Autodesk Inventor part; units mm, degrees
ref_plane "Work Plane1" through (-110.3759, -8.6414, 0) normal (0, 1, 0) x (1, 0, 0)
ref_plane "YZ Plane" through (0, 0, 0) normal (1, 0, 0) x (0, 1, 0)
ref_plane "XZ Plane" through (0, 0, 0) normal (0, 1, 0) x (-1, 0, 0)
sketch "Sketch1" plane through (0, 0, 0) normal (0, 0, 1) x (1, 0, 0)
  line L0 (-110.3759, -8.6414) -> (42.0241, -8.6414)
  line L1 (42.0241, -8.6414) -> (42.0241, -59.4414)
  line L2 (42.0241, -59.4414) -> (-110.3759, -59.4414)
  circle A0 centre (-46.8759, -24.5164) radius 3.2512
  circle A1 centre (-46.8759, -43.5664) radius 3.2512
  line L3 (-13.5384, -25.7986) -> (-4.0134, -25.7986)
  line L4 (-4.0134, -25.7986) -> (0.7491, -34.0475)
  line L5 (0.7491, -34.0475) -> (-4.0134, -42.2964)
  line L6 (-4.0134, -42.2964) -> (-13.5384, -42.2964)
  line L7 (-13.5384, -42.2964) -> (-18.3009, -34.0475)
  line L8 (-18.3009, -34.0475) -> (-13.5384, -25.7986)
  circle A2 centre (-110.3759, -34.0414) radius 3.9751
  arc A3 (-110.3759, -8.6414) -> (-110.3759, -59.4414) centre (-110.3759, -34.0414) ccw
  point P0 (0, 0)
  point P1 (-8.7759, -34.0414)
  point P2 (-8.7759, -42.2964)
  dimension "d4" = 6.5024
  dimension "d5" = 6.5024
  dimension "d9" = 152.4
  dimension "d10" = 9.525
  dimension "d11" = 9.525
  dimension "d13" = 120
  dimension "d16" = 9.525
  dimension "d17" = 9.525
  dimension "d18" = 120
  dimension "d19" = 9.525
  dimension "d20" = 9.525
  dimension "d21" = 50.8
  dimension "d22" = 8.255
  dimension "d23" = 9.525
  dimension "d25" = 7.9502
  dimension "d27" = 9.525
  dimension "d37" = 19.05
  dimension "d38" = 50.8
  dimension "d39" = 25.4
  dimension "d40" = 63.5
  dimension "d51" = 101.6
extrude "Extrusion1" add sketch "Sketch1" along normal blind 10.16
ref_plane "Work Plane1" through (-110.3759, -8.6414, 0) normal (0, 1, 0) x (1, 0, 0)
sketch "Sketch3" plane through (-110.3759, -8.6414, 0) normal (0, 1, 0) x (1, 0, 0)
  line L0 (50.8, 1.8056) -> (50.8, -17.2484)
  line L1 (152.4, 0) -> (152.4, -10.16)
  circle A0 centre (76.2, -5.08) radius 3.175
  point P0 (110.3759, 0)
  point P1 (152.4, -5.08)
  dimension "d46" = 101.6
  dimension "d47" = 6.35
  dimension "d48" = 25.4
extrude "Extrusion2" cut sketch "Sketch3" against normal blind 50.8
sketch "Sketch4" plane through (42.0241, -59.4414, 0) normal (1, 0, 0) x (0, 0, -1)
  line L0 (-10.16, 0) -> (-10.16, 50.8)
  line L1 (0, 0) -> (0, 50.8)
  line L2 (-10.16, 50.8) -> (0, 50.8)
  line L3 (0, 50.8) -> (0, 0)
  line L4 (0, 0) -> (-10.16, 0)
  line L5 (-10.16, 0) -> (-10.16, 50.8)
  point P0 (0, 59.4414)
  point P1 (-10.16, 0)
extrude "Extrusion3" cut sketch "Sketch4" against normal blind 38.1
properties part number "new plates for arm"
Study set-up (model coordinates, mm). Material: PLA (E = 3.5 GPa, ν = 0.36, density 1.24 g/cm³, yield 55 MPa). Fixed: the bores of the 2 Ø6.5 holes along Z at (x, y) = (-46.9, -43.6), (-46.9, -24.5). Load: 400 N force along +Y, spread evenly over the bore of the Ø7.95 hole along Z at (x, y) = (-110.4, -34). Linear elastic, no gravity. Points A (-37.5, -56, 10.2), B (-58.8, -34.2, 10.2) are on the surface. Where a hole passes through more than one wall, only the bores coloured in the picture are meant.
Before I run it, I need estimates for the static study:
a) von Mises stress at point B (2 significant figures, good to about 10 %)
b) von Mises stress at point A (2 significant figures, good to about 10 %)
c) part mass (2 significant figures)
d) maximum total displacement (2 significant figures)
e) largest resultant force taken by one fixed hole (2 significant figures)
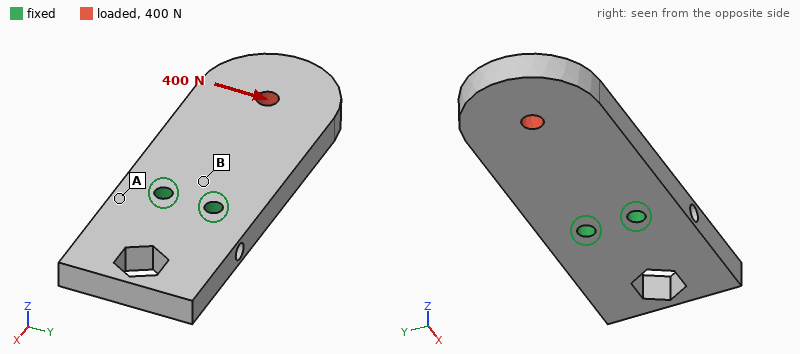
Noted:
3.9 MPa
1.7 MPa
79 g
0.28 mm
1.1 kN
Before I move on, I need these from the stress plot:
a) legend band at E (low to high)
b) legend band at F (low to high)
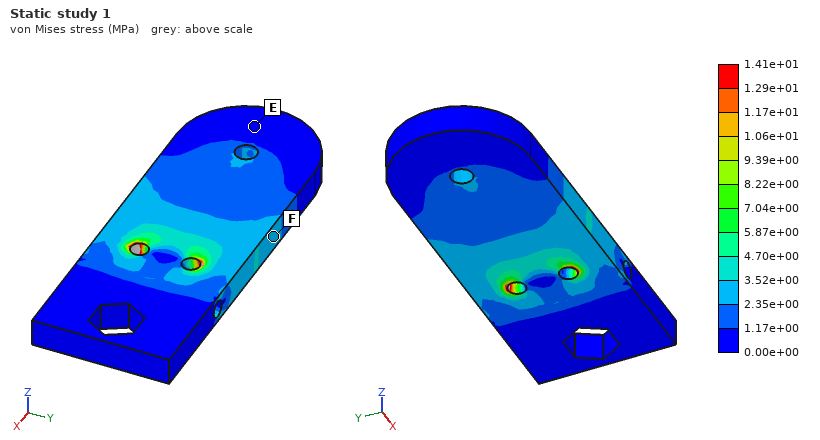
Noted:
0.00e+00 to 1.17e+00 MPa
2.35e+00 to 3.52e+00 MPa
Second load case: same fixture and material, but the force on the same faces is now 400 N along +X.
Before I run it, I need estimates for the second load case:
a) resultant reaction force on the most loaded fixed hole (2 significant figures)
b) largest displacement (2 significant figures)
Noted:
200 N
21 µm
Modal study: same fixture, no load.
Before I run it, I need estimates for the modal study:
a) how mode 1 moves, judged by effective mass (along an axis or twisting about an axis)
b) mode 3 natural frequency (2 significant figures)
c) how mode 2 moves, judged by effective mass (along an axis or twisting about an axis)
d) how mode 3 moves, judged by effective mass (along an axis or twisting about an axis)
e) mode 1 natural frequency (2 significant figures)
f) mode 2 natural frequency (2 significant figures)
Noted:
along Z
1200 Hz
along Z
along Y
400 Hz
1100 Hz
